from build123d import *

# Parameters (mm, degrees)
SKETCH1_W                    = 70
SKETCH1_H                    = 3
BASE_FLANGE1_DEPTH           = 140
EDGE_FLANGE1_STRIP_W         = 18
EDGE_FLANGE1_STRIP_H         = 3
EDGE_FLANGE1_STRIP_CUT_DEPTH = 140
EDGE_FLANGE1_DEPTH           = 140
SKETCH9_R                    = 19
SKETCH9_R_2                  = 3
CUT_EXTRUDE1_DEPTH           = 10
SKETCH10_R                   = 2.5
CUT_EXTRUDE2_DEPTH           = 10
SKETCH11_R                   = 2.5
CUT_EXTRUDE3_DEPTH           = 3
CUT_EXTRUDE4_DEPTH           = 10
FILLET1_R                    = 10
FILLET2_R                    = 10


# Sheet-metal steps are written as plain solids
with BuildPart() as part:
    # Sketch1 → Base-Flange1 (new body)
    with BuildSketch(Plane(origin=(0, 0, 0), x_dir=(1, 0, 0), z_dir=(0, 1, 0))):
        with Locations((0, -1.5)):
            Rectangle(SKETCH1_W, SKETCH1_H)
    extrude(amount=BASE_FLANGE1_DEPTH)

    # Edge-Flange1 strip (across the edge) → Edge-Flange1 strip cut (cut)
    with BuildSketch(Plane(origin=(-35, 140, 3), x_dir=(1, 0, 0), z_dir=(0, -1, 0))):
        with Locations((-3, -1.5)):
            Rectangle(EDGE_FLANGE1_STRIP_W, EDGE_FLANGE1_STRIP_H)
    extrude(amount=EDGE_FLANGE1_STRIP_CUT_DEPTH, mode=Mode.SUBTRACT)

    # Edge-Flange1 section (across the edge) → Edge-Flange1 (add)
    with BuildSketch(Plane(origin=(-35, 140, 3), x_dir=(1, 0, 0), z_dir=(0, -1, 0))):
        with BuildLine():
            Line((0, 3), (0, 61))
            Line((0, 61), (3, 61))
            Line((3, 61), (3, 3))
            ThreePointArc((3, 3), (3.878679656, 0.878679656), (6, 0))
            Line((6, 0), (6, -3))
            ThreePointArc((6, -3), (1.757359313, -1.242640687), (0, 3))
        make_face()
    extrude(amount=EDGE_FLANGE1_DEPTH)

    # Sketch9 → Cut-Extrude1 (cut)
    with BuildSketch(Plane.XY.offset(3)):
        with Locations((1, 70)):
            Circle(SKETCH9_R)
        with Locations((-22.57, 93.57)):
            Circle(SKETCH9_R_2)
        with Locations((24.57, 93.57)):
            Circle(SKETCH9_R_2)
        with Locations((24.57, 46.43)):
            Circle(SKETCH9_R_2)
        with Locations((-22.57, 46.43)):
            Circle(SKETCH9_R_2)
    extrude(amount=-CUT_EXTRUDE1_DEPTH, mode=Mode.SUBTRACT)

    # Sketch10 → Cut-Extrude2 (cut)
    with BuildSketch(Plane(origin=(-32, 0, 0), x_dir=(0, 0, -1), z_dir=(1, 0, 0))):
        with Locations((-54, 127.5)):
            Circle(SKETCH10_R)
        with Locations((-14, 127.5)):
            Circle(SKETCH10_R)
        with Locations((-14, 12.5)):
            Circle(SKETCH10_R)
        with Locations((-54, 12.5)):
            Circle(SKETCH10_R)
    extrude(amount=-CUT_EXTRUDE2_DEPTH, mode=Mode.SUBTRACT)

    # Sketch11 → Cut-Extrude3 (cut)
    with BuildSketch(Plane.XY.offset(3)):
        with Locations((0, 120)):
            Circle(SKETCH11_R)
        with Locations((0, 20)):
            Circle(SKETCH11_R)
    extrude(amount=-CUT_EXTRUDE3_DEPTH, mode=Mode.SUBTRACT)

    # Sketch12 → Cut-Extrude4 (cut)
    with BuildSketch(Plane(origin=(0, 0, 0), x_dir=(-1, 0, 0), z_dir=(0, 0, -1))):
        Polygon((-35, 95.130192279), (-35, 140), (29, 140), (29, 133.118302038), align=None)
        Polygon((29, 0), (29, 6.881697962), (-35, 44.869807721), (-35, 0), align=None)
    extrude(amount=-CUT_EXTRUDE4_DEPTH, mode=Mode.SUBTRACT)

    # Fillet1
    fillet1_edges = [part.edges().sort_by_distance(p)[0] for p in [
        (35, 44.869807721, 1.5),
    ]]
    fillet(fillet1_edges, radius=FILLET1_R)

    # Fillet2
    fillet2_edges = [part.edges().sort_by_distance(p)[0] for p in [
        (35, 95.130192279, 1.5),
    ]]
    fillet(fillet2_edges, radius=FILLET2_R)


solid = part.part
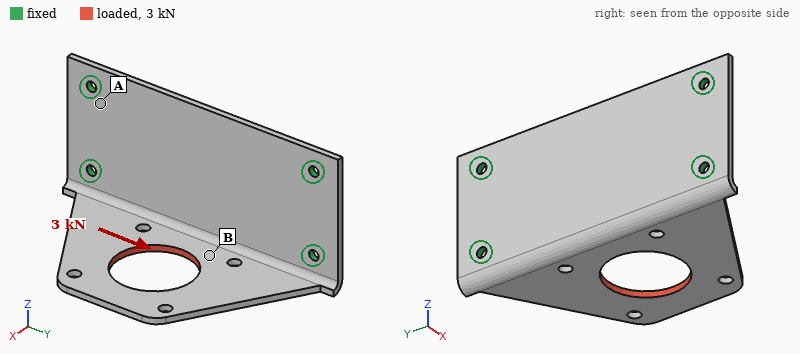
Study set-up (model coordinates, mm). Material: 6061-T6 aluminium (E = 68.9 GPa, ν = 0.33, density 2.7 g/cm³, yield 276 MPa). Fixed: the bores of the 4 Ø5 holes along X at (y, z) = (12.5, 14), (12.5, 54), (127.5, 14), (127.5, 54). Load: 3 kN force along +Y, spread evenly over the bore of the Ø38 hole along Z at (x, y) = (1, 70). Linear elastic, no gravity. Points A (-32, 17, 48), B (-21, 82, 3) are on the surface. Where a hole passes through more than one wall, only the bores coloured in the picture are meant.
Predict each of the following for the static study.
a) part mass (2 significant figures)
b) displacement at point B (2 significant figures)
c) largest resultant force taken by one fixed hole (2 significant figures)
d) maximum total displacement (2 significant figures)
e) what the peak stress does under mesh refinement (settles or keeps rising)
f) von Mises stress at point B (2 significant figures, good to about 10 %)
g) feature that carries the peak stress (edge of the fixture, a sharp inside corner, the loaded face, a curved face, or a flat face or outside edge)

110 g
0.041 mm
1.6 kN
0.24 mm
keeps rising
39 MPa
edge of the fixture
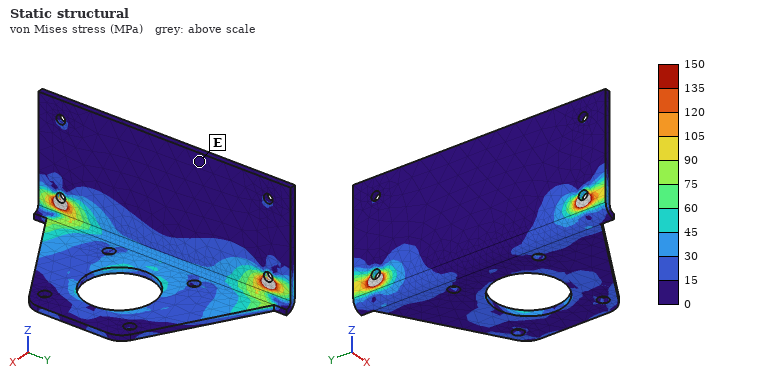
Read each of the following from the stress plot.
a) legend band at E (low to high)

0 to 15 MPa
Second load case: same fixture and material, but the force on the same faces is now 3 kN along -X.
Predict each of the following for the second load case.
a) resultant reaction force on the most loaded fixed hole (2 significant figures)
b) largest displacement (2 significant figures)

2.0 kN
1.0 mm
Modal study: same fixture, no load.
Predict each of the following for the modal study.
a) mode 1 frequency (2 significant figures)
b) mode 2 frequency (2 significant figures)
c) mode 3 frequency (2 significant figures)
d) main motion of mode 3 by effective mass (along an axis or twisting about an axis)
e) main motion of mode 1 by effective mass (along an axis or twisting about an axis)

520 Hz
1300 Hz
1500 Hz
along X
along Z
